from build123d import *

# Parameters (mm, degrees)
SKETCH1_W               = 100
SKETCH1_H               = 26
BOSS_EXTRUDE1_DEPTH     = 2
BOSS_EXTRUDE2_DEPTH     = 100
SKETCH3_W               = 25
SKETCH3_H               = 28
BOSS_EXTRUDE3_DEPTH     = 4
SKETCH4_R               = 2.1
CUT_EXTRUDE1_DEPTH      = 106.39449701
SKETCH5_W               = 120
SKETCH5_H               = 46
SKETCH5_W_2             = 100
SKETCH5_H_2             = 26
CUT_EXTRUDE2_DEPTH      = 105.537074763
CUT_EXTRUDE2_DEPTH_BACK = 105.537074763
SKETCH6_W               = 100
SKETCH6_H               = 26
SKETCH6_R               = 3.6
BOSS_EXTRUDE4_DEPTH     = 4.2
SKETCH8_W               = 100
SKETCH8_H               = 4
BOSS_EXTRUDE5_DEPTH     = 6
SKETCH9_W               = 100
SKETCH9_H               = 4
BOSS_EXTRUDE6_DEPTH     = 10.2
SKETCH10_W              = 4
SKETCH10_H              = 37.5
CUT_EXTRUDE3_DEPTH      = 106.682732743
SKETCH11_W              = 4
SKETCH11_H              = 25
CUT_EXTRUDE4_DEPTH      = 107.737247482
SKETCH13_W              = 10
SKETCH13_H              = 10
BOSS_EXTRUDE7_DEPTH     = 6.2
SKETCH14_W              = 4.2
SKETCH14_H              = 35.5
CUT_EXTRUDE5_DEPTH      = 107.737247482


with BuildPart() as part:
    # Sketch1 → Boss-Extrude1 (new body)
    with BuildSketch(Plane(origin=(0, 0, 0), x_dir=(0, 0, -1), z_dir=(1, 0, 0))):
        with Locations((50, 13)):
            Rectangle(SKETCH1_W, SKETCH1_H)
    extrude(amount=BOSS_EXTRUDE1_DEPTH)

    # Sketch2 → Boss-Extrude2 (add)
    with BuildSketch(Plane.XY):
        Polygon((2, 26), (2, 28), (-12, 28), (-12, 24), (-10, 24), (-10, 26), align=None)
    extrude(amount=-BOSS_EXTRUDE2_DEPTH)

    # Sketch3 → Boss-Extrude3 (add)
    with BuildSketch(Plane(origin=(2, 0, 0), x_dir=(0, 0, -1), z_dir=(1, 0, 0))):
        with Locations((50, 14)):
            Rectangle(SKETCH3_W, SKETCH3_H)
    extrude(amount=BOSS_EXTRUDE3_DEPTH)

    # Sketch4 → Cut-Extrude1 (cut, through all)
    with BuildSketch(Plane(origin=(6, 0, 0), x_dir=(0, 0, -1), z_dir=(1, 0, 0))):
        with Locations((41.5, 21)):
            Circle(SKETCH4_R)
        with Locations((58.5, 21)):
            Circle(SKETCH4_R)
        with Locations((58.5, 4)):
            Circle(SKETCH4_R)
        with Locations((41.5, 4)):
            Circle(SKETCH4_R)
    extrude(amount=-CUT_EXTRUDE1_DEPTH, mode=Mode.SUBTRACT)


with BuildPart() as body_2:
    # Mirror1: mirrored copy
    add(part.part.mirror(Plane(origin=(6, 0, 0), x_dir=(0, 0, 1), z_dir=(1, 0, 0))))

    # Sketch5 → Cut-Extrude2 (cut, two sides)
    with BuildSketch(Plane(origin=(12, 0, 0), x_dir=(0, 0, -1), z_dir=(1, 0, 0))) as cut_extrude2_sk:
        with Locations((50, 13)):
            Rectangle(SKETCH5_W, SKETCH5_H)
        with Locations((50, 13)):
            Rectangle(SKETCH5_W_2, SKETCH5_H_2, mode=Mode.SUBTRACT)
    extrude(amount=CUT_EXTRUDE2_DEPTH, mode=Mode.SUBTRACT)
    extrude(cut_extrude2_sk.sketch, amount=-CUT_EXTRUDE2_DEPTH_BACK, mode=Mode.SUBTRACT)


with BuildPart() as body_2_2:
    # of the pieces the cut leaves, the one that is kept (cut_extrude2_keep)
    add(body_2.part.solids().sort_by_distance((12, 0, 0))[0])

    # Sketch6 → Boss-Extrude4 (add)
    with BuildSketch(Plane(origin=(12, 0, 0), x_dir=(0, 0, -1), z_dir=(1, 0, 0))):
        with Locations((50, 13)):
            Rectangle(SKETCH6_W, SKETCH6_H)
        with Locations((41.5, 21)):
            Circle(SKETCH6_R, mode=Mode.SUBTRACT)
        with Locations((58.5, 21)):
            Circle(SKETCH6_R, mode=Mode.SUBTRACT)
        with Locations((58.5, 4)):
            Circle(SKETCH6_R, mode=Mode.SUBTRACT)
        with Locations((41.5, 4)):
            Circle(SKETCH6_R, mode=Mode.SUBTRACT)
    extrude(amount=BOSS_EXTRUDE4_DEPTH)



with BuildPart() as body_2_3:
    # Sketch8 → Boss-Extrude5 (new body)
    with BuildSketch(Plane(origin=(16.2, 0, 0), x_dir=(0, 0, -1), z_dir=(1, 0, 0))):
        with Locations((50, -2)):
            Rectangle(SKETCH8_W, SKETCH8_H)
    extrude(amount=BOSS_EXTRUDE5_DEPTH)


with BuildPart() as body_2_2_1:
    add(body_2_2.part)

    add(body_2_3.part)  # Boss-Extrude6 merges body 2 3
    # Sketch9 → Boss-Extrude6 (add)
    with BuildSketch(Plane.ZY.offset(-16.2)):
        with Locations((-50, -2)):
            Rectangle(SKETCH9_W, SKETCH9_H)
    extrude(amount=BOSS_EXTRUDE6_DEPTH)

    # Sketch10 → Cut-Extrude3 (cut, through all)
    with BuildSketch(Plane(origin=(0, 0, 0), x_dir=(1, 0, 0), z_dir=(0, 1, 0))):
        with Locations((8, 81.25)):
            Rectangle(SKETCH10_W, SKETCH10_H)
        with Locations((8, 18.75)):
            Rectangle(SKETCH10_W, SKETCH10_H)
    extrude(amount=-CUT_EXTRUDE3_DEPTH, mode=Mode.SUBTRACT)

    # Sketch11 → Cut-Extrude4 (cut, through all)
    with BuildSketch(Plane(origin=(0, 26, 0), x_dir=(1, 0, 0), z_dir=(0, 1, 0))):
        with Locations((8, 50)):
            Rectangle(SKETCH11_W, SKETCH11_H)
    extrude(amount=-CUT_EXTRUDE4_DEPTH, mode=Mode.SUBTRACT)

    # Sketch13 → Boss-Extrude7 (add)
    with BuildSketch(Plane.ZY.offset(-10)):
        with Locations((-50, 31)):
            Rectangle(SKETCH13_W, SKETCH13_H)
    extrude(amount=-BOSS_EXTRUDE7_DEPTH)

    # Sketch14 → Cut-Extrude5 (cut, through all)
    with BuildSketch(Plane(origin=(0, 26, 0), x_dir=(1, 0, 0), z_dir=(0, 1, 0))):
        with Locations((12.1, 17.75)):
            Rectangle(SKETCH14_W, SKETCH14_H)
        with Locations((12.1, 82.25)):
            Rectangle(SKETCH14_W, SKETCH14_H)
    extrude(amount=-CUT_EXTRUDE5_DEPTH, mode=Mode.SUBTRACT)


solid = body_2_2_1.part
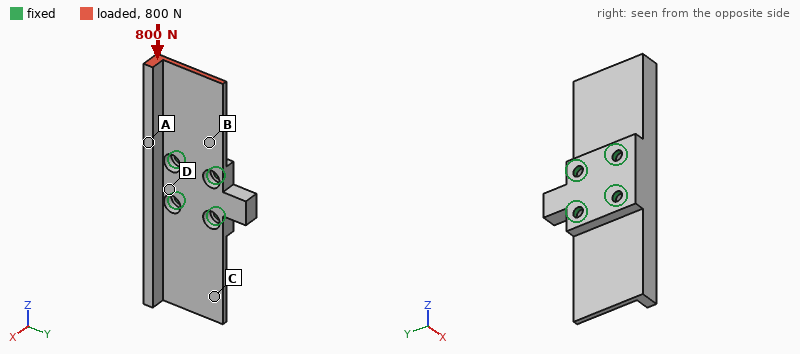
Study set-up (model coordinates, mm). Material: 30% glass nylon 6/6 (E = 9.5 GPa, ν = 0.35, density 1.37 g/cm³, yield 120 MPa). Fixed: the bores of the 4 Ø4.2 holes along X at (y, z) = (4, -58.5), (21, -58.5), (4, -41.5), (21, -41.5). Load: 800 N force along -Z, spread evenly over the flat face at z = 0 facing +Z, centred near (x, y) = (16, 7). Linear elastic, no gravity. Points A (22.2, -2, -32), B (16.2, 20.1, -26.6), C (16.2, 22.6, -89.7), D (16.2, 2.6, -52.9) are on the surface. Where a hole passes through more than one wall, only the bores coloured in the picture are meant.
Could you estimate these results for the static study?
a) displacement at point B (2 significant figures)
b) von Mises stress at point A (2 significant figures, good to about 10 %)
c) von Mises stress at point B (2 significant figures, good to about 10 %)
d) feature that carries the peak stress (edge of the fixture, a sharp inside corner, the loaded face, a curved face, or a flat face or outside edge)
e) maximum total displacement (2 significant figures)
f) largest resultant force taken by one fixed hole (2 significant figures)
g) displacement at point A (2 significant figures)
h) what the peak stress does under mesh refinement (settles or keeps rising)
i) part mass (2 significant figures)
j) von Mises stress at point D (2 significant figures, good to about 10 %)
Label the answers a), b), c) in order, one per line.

a) 0.059 mm
b) 10 MPa
c) 8.7 MPa
d) edge of the fixture
e) 0.14 mm
f) 330 N
g) 0.052 mm
h) keeps rising
i) 16 g
j) 5.1 MPa
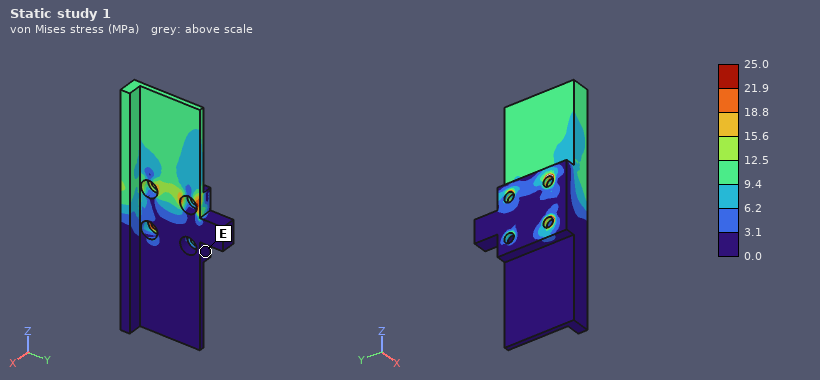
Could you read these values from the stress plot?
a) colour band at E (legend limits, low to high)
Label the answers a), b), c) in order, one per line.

a) 0.0 to 3.1 MPa
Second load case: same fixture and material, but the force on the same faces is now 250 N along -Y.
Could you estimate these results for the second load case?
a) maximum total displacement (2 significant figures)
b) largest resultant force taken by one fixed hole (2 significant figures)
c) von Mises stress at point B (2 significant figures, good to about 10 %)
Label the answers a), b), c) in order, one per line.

a) 0.44 mm
b) 350 N
c) 13 MPa
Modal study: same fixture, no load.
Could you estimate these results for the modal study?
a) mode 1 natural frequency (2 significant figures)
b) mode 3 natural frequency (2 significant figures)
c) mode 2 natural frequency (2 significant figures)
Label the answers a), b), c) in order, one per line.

a) 1200 Hz
b) 2100 Hz
c) 1200 Hz
